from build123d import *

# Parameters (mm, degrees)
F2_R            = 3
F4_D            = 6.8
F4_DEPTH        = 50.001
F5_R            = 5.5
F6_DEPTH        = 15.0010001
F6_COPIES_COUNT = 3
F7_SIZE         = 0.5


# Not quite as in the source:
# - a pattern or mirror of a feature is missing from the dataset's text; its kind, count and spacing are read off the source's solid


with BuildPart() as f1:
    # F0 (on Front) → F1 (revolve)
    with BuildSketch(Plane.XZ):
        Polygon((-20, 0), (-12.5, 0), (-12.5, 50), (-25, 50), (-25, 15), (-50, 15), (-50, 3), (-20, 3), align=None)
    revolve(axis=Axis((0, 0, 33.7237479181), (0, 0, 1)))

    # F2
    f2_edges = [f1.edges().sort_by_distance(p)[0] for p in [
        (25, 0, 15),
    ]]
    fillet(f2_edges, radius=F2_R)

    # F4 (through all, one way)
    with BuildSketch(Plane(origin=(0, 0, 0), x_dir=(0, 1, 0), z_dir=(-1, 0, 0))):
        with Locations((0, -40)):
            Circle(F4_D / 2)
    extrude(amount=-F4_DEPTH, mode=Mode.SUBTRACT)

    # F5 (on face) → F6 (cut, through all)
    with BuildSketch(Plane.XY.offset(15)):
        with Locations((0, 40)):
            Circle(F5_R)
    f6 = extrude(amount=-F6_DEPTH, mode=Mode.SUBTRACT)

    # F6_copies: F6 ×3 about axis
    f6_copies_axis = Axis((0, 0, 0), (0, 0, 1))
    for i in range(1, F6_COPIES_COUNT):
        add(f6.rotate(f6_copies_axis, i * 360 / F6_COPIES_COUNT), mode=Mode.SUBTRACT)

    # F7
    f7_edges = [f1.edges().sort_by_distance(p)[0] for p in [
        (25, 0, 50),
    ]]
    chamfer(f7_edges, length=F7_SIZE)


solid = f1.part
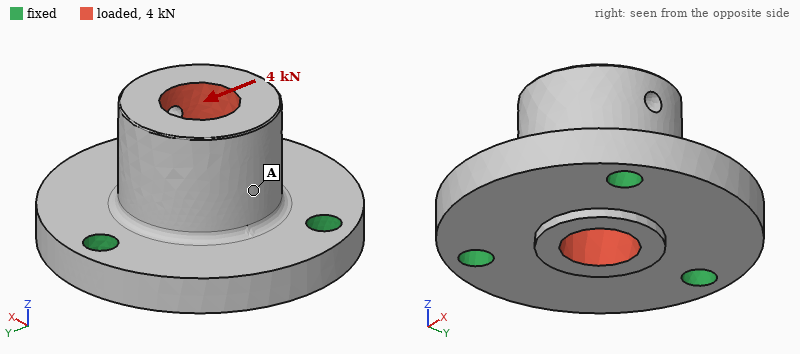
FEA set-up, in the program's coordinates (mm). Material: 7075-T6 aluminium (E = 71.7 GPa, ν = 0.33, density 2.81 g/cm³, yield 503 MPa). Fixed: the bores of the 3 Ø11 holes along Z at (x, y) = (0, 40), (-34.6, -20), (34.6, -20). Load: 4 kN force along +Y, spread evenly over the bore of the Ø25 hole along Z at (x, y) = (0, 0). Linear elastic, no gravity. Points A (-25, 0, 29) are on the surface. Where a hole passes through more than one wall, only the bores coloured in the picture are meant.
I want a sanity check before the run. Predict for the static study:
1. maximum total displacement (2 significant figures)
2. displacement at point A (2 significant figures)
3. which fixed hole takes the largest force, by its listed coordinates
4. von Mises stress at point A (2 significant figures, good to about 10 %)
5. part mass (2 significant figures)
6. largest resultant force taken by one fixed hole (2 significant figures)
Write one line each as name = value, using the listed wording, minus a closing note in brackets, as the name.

maximum total displacement = 9.3 µm
displacement at point A = 4.4 µm
which fixed hole takes the largest force, by its listed coordinates = (0, 40)
von Mises stress at point A = 2.4 MPa
part mass = 390 g
largest resultant force taken by one fixed hole = 1.9 kN
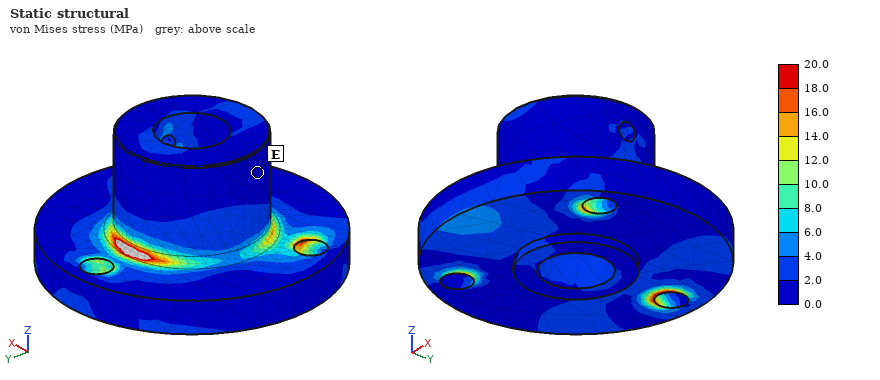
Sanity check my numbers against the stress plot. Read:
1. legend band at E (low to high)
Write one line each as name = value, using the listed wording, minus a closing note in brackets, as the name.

legend band at E = 0.0 to 2.0 MPa
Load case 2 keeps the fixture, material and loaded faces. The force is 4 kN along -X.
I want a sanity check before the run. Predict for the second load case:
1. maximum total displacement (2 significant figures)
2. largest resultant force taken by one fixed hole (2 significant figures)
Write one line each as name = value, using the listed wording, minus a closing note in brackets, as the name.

maximum total displacement = 9.0 µm
largest resultant force taken by one fixed hole = 1.7 kN
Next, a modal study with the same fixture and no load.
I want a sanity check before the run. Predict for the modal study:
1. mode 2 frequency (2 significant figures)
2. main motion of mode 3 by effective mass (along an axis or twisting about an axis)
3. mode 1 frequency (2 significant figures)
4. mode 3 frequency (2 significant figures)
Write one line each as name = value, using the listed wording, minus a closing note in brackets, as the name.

mode 2 frequency = 7500 Hz
main motion of mode 3 by effective mass = along Z
mode 1 frequency = 7500 Hz
mode 3 frequency = 8800 Hz
